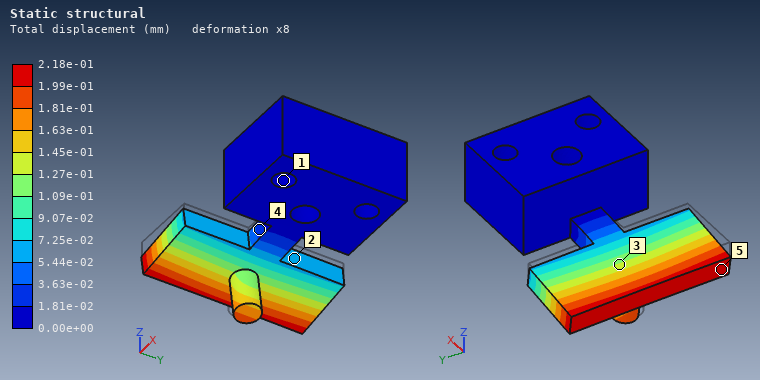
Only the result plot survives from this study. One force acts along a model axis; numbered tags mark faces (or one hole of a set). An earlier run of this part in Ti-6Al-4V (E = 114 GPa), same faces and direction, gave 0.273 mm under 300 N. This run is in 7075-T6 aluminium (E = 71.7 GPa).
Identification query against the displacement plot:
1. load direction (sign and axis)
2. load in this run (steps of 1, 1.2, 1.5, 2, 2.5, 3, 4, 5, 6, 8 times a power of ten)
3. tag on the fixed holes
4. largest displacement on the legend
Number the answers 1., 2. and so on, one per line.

1. -Z
2. 150 N
3. 1
4. 2.18e-01 mm
